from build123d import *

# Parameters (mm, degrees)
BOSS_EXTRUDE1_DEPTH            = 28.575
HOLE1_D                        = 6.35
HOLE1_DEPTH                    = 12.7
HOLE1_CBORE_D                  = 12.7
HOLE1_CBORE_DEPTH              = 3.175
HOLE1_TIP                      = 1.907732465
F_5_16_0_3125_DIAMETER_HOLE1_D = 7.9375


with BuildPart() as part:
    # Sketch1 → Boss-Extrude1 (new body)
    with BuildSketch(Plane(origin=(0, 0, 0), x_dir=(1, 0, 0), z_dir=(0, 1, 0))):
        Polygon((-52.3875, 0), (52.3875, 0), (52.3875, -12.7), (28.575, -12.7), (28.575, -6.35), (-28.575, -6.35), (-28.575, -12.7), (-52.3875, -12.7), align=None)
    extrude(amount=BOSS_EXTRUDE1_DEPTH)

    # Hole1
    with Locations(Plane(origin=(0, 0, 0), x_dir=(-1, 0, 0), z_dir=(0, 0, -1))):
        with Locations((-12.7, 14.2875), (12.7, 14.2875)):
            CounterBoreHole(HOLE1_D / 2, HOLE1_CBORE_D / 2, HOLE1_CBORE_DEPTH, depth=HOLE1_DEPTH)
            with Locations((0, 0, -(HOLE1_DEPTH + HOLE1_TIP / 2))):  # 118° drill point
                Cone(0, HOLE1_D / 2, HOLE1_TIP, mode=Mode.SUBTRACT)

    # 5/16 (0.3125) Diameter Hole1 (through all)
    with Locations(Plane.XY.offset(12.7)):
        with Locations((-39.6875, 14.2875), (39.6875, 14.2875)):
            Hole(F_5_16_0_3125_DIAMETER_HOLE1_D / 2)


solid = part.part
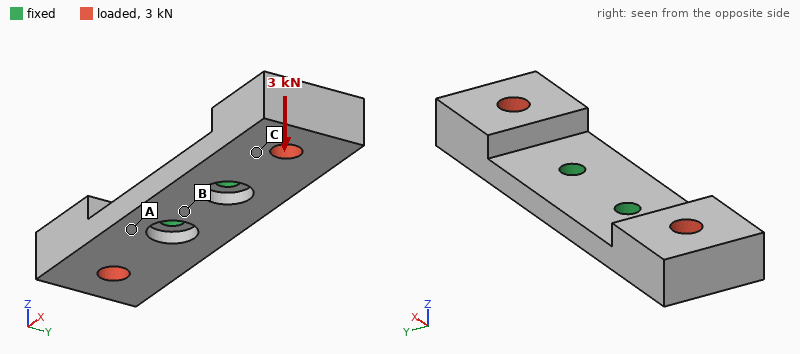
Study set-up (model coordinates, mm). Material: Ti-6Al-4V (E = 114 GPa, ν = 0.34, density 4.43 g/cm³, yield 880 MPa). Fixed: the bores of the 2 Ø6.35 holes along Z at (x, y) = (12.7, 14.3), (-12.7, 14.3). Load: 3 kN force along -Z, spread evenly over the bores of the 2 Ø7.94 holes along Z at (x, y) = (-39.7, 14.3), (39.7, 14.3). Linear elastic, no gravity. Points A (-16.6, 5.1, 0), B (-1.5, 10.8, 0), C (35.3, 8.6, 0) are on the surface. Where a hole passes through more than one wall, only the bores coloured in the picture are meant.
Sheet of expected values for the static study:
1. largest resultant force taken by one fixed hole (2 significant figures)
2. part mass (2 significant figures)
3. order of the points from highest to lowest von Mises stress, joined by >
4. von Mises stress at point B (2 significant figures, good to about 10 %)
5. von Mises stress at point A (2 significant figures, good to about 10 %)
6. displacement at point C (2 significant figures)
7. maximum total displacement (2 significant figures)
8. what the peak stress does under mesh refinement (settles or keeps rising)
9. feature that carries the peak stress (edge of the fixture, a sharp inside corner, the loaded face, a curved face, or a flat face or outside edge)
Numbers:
4.3 kN
110 g
A > B > C
79 MPa
220 MPa
0.19 mm
0.37 mm
keeps rising
edge of the fixture
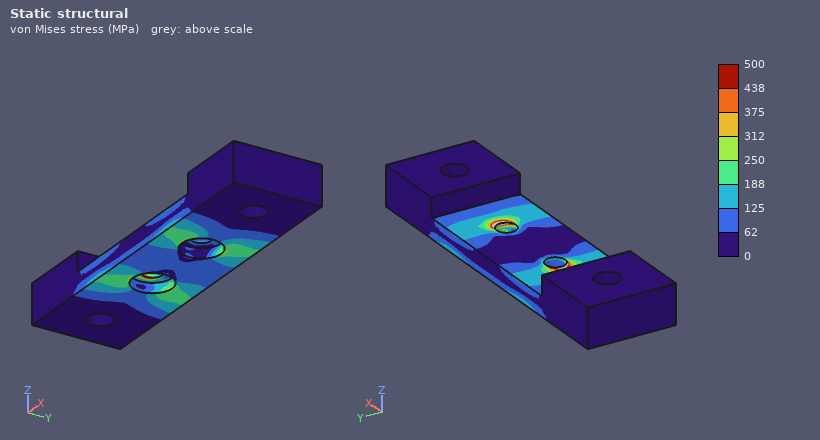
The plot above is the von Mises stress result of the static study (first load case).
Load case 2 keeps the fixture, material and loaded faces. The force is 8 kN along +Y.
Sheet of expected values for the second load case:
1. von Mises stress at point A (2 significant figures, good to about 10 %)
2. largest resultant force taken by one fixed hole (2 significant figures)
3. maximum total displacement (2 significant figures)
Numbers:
81 MPa
4.0 kN
0.11 mm
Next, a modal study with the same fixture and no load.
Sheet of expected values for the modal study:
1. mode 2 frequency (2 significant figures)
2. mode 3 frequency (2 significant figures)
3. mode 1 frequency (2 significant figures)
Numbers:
2000 Hz
4700 Hz
1900 Hz
